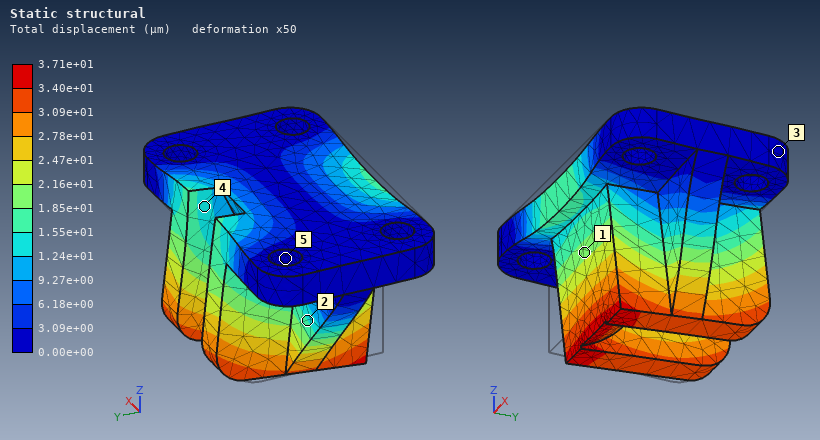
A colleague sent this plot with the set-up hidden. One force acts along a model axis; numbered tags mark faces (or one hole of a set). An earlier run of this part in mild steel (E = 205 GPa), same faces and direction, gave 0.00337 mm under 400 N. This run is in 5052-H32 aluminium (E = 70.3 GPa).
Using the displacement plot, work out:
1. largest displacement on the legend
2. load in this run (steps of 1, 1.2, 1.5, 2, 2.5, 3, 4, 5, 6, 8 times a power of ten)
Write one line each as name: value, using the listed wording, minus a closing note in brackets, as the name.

largest displacement on the legend: 3.71e+01 µm
load in this run: 1.5 kN
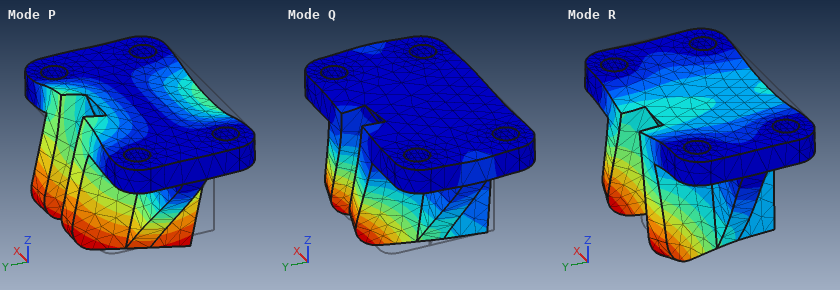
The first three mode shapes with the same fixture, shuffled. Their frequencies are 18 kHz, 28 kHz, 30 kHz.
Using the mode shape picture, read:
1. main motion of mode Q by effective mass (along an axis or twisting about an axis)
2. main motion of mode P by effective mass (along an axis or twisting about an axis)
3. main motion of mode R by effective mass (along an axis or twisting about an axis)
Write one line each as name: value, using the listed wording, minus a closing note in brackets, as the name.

main motion of mode Q by effective mass: along X
main motion of mode P by effective mass: along Y
main motion of mode R by effective mass: along Z
